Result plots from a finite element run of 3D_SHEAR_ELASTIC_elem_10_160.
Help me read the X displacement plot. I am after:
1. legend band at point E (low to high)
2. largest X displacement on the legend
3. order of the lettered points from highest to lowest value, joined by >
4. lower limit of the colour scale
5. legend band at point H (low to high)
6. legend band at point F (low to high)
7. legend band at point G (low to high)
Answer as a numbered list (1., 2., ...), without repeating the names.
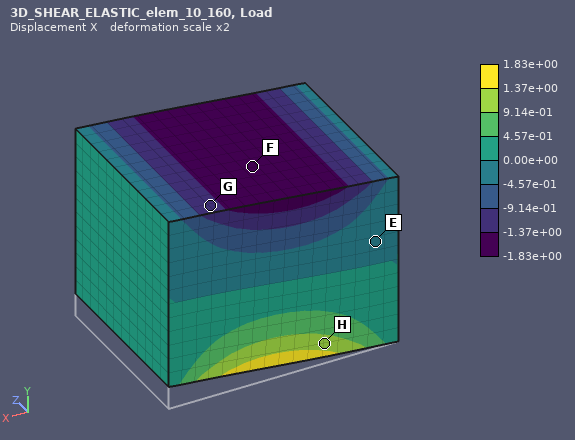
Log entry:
1. -4.57e-01 to 0.00e+00
2. 1.83e+00
3. H > E > G > F
4. -1.83e+00
5. 9.14e-01 to 1.37e+00
6. -1.83e+00 to -1.37e+00
7. -1.37e+00 to -9.14e-01
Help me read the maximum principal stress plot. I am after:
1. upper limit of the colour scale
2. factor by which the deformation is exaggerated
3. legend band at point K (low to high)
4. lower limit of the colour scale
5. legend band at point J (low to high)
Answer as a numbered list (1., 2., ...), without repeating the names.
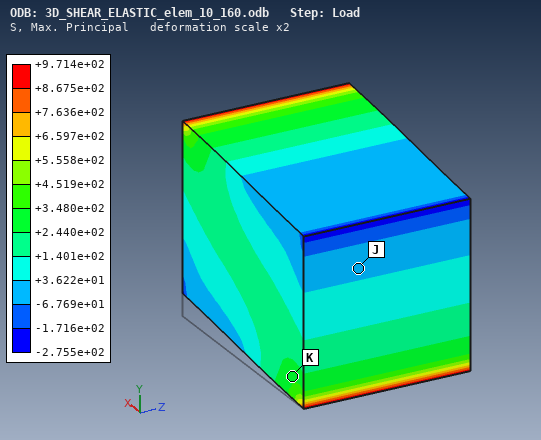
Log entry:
1. +9.714e+02
2. 2
3. +2.440e+02 to +3.480e+02
4. -2.755e+02
5. -6.769e+01 to +3.622e+01
